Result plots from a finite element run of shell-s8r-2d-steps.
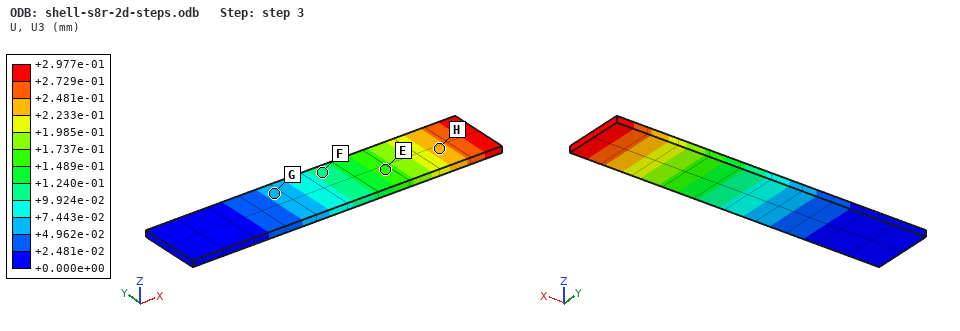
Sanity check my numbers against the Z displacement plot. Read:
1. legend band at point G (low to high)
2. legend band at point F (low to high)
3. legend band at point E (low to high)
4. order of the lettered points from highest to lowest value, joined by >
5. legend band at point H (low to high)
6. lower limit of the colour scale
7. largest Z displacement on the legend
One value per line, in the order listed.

+4.962e-02 to +7.443e-02 mm
+9.924e-02 to +1.240e-01 mm
+1.489e-01 to +1.737e-01 mm
H > E > F > G
+2.233e-01 to +2.481e-01 mm
+0.000e+00 mm
+2.977e-01 mm
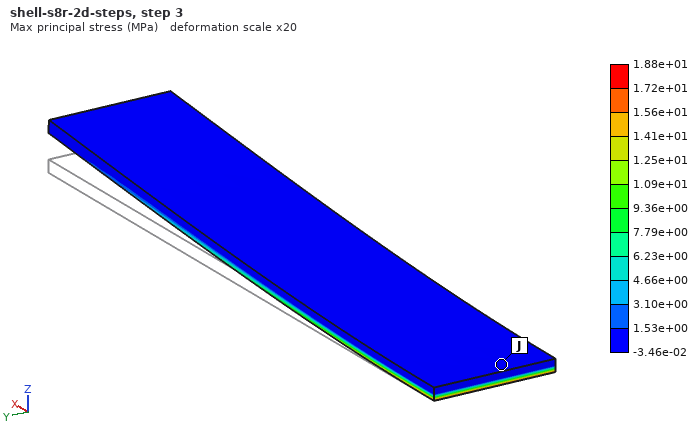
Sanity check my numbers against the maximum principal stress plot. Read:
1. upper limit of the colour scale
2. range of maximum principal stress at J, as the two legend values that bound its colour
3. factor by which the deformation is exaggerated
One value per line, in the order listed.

1.88e+01 MPa
-3.46e-02 to 1.53e+00 MPa
20
